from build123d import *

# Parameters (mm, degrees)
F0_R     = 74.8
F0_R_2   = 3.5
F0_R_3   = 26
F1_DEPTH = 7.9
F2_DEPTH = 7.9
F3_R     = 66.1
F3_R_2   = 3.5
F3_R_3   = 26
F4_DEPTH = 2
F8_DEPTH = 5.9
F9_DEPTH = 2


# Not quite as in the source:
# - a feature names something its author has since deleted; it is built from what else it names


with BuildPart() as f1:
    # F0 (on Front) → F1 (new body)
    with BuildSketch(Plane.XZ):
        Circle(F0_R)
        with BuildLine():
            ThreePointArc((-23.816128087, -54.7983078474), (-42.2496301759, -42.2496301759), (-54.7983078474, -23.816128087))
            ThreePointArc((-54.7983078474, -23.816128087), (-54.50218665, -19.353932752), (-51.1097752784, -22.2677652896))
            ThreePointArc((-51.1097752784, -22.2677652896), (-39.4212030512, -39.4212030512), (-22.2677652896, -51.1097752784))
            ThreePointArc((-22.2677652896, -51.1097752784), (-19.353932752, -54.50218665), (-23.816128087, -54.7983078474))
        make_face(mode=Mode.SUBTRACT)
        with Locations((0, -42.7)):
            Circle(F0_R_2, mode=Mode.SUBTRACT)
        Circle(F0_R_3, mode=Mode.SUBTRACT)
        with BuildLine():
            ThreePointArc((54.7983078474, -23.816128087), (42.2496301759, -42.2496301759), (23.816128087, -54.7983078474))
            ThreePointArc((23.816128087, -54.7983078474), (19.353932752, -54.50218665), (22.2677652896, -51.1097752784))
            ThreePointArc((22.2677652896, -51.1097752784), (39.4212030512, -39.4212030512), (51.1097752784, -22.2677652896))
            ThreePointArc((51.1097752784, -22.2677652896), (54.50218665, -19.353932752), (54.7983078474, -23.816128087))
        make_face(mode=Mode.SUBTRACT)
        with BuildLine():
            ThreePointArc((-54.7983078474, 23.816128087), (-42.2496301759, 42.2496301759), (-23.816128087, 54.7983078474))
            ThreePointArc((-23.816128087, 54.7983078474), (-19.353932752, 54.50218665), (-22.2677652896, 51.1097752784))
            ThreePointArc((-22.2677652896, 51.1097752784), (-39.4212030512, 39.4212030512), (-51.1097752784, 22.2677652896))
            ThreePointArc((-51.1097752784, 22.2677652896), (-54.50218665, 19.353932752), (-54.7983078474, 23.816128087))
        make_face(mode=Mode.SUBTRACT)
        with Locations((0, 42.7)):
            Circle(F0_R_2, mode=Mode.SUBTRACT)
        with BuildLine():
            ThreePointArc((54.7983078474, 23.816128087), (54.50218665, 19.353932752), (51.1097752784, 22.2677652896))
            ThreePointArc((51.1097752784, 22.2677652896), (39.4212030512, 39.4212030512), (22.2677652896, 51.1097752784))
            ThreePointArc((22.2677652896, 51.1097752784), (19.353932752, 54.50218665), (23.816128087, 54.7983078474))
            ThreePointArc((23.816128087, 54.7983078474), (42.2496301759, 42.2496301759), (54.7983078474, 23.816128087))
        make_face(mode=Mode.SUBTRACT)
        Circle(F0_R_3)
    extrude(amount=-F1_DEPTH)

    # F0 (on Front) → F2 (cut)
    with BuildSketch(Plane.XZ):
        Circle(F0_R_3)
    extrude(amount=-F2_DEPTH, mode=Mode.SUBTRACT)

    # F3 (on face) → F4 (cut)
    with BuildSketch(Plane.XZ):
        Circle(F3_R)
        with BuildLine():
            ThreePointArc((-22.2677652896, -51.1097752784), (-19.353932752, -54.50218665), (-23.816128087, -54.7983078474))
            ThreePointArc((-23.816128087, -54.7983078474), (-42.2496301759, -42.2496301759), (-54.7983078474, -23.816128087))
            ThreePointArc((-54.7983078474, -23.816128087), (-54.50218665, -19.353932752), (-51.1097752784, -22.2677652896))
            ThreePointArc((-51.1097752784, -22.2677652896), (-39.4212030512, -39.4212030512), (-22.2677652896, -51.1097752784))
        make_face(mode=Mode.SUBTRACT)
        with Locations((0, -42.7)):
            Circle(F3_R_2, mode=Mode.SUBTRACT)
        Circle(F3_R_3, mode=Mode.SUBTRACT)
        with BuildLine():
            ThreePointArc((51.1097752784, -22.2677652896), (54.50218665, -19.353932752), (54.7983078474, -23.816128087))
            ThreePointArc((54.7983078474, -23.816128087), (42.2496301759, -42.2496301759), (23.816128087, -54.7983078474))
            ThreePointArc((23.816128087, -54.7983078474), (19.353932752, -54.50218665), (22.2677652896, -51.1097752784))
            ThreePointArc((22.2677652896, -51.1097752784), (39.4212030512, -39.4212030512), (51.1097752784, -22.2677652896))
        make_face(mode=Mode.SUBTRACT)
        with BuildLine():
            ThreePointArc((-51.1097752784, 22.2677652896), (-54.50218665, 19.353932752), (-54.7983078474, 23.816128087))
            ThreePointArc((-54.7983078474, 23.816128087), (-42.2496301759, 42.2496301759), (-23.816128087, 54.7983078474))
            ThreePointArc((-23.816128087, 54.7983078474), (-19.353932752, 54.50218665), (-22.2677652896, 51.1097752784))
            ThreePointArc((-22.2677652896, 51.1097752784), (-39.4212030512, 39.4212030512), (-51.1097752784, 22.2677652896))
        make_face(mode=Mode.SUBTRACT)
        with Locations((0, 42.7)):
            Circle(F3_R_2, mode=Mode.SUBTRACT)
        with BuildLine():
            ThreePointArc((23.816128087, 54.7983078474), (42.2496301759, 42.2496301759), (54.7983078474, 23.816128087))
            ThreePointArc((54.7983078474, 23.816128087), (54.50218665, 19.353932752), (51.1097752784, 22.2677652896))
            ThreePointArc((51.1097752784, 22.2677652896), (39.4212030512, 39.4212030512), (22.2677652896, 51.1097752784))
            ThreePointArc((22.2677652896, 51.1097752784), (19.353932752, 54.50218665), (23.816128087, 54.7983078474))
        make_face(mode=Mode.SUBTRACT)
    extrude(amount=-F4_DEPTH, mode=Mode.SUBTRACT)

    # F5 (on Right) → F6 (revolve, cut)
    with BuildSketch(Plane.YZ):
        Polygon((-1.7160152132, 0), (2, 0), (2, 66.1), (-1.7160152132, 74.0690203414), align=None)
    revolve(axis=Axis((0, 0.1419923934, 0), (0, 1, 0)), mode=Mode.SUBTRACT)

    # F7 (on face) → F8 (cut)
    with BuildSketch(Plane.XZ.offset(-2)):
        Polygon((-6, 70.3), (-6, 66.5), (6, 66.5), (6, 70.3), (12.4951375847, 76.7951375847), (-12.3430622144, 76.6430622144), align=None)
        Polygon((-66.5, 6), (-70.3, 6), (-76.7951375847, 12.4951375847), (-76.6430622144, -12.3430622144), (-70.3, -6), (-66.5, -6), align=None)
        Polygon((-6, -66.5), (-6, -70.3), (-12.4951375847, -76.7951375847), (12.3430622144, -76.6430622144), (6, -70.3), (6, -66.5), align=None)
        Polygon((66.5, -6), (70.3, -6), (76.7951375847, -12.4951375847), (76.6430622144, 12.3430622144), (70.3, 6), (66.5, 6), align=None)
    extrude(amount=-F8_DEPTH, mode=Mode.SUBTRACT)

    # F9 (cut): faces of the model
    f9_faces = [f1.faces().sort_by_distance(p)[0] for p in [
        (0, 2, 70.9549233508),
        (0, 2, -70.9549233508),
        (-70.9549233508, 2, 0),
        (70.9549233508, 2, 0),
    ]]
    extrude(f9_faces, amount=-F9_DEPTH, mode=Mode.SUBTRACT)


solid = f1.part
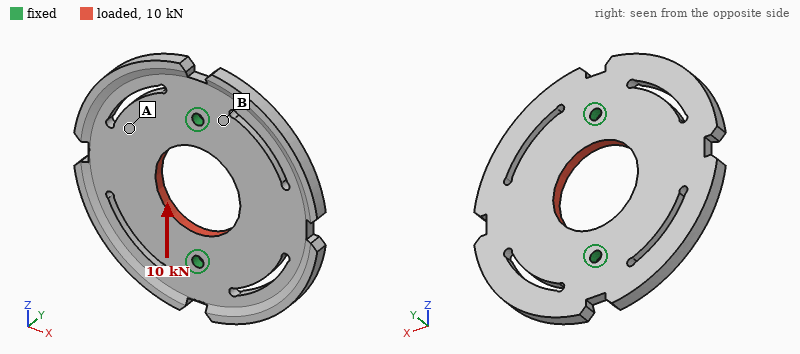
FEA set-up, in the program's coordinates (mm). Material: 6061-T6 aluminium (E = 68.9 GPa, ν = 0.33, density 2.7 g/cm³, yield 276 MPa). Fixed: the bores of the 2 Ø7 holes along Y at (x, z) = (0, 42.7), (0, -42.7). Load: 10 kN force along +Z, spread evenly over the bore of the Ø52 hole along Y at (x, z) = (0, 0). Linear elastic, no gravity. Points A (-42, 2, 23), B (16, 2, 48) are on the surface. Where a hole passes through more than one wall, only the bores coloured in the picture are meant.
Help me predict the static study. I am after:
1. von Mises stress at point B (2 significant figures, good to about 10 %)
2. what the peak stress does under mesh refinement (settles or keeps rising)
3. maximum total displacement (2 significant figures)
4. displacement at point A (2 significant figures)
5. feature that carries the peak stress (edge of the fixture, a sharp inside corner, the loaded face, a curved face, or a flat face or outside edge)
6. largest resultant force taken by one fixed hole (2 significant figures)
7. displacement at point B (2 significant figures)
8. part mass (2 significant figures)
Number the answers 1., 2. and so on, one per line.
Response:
1. 12 MPa
2. keeps rising
3. 19 µm
4. 15 µm
5. edge of the fixture
6. 5.0 kN
7. 7.0 µm
8. 240 g
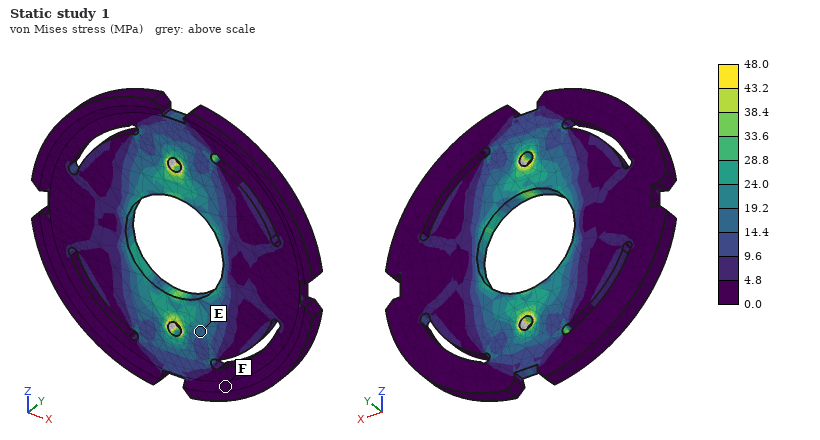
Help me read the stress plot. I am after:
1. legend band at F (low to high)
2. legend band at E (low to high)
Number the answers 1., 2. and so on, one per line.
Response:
1. 0.0 to 4.8 MPa
2. 14.4 to 19.2 MPa
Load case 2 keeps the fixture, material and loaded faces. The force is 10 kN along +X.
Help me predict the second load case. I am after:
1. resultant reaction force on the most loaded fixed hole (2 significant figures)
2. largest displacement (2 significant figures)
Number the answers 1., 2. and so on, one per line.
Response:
1. 5.0 kN
2. 17 µm
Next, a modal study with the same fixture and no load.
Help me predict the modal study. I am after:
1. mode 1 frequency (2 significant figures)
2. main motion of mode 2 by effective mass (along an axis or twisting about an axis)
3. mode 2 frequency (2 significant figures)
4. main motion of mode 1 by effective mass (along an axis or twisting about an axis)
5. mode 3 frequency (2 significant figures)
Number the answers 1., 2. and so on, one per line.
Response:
1. 840 Hz
2. along Y
3. 920 Hz
4. twisting about Z
5. 1800 Hz
